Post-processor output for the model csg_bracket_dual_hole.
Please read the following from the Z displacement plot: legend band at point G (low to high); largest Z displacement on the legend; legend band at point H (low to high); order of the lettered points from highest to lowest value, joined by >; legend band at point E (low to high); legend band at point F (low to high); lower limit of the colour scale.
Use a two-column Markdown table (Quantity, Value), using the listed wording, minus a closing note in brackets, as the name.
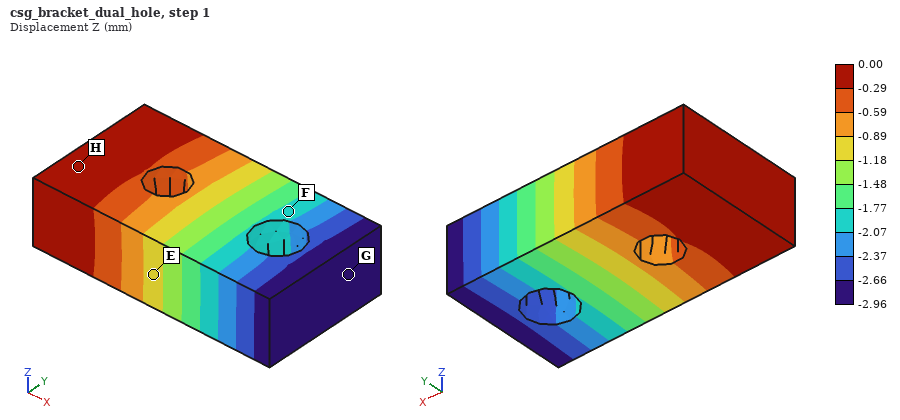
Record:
| Quantity | Value |
|---|---|
| legend band at point G | -2.96 to -2.66 mm |
| largest Z displacement on the legend | 0.00 mm |
| legend band at point H | -0.29 to 0.00 mm |
| order of the lettered points from highest to lowest value, joined by > | H > E > F > G |
| legend band at point E | -1.18 to -0.89 mm |
| legend band at point F | -2.07 to -1.77 mm |
| lower limit of the colour scale | -2.96 mm |
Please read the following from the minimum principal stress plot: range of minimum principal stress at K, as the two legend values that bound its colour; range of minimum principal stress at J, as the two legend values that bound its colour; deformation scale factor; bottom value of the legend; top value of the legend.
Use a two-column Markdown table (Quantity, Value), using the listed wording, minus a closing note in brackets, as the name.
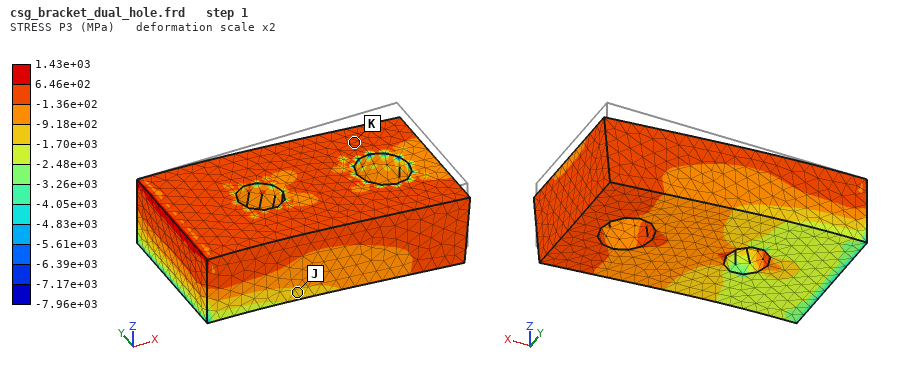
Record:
| Quantity | Value |
|---|---|
| range of minimum principal stress at K, as the two legend values that bound its colour | -1.36e+02 to 6.46e+02 MPa |
| range of minimum principal stress at J, as the two legend values that bound its colour | -1.70e+03 to -9.18e+02 MPa |
| deformation scale factor | 2 |
| bottom value of the legend | -7.96e+03 MPa |
| top value of the legend | 1.43e+03 MPa |
